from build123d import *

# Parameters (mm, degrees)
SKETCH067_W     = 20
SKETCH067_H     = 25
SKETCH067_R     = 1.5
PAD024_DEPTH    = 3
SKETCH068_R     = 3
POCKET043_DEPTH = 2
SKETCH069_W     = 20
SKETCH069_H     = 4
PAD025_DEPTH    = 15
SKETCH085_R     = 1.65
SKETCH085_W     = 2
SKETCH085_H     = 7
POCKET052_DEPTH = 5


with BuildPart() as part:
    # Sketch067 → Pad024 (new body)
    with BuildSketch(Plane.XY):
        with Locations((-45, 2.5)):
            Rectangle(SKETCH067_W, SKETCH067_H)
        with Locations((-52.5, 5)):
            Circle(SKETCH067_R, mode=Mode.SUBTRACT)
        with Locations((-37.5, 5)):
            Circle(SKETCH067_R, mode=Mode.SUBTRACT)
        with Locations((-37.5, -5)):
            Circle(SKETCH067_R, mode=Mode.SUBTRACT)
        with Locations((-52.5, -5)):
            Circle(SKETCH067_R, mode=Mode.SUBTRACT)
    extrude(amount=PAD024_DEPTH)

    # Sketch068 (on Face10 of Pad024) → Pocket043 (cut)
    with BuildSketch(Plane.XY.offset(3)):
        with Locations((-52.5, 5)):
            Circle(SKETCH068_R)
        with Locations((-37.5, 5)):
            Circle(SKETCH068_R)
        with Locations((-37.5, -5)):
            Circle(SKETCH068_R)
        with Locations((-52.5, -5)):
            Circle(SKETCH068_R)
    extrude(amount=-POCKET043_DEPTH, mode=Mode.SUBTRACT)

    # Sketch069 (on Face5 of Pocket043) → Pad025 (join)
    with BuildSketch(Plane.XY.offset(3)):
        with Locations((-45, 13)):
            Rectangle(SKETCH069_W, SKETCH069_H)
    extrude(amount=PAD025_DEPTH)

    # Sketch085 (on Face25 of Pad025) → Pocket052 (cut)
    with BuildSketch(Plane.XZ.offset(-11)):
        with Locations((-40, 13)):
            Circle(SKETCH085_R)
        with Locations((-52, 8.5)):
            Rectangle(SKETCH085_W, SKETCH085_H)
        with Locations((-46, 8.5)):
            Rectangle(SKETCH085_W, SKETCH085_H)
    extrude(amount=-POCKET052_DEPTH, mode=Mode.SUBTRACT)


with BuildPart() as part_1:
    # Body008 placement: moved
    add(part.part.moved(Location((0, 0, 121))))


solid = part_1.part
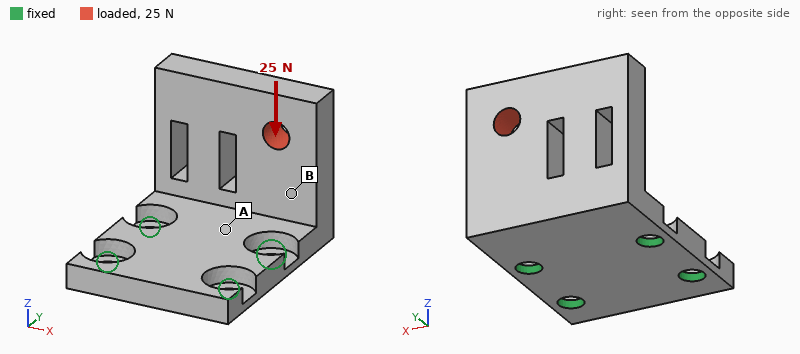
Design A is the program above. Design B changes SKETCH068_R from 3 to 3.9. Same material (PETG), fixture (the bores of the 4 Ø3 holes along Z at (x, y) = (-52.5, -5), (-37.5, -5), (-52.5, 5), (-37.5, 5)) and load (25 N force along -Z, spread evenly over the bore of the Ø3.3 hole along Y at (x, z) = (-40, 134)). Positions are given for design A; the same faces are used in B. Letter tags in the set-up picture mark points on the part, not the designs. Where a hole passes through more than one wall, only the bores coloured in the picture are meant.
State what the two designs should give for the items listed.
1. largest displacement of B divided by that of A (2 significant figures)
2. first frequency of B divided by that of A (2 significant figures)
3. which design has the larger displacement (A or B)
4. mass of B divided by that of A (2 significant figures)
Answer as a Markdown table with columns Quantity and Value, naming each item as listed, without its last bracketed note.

| Quantity | Value |
|---|---|
| largest displacement of B divided by that of A | 1.2 |
| first frequency of B divided by that of A | 0.91 |
| which design has the larger displacement | B |
| mass of B divided by that of A | 0.95 |
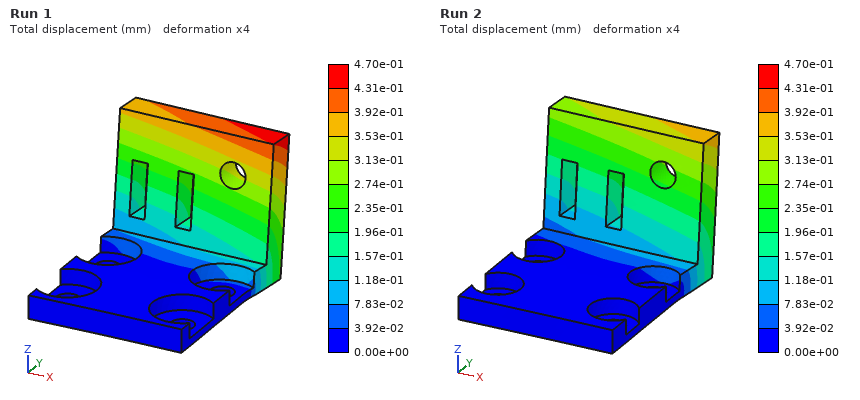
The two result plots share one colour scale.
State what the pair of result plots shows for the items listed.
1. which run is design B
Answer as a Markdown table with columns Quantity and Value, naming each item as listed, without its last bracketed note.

| Quantity | Value |
|---|---|
| which run is design B | Run 1 |
